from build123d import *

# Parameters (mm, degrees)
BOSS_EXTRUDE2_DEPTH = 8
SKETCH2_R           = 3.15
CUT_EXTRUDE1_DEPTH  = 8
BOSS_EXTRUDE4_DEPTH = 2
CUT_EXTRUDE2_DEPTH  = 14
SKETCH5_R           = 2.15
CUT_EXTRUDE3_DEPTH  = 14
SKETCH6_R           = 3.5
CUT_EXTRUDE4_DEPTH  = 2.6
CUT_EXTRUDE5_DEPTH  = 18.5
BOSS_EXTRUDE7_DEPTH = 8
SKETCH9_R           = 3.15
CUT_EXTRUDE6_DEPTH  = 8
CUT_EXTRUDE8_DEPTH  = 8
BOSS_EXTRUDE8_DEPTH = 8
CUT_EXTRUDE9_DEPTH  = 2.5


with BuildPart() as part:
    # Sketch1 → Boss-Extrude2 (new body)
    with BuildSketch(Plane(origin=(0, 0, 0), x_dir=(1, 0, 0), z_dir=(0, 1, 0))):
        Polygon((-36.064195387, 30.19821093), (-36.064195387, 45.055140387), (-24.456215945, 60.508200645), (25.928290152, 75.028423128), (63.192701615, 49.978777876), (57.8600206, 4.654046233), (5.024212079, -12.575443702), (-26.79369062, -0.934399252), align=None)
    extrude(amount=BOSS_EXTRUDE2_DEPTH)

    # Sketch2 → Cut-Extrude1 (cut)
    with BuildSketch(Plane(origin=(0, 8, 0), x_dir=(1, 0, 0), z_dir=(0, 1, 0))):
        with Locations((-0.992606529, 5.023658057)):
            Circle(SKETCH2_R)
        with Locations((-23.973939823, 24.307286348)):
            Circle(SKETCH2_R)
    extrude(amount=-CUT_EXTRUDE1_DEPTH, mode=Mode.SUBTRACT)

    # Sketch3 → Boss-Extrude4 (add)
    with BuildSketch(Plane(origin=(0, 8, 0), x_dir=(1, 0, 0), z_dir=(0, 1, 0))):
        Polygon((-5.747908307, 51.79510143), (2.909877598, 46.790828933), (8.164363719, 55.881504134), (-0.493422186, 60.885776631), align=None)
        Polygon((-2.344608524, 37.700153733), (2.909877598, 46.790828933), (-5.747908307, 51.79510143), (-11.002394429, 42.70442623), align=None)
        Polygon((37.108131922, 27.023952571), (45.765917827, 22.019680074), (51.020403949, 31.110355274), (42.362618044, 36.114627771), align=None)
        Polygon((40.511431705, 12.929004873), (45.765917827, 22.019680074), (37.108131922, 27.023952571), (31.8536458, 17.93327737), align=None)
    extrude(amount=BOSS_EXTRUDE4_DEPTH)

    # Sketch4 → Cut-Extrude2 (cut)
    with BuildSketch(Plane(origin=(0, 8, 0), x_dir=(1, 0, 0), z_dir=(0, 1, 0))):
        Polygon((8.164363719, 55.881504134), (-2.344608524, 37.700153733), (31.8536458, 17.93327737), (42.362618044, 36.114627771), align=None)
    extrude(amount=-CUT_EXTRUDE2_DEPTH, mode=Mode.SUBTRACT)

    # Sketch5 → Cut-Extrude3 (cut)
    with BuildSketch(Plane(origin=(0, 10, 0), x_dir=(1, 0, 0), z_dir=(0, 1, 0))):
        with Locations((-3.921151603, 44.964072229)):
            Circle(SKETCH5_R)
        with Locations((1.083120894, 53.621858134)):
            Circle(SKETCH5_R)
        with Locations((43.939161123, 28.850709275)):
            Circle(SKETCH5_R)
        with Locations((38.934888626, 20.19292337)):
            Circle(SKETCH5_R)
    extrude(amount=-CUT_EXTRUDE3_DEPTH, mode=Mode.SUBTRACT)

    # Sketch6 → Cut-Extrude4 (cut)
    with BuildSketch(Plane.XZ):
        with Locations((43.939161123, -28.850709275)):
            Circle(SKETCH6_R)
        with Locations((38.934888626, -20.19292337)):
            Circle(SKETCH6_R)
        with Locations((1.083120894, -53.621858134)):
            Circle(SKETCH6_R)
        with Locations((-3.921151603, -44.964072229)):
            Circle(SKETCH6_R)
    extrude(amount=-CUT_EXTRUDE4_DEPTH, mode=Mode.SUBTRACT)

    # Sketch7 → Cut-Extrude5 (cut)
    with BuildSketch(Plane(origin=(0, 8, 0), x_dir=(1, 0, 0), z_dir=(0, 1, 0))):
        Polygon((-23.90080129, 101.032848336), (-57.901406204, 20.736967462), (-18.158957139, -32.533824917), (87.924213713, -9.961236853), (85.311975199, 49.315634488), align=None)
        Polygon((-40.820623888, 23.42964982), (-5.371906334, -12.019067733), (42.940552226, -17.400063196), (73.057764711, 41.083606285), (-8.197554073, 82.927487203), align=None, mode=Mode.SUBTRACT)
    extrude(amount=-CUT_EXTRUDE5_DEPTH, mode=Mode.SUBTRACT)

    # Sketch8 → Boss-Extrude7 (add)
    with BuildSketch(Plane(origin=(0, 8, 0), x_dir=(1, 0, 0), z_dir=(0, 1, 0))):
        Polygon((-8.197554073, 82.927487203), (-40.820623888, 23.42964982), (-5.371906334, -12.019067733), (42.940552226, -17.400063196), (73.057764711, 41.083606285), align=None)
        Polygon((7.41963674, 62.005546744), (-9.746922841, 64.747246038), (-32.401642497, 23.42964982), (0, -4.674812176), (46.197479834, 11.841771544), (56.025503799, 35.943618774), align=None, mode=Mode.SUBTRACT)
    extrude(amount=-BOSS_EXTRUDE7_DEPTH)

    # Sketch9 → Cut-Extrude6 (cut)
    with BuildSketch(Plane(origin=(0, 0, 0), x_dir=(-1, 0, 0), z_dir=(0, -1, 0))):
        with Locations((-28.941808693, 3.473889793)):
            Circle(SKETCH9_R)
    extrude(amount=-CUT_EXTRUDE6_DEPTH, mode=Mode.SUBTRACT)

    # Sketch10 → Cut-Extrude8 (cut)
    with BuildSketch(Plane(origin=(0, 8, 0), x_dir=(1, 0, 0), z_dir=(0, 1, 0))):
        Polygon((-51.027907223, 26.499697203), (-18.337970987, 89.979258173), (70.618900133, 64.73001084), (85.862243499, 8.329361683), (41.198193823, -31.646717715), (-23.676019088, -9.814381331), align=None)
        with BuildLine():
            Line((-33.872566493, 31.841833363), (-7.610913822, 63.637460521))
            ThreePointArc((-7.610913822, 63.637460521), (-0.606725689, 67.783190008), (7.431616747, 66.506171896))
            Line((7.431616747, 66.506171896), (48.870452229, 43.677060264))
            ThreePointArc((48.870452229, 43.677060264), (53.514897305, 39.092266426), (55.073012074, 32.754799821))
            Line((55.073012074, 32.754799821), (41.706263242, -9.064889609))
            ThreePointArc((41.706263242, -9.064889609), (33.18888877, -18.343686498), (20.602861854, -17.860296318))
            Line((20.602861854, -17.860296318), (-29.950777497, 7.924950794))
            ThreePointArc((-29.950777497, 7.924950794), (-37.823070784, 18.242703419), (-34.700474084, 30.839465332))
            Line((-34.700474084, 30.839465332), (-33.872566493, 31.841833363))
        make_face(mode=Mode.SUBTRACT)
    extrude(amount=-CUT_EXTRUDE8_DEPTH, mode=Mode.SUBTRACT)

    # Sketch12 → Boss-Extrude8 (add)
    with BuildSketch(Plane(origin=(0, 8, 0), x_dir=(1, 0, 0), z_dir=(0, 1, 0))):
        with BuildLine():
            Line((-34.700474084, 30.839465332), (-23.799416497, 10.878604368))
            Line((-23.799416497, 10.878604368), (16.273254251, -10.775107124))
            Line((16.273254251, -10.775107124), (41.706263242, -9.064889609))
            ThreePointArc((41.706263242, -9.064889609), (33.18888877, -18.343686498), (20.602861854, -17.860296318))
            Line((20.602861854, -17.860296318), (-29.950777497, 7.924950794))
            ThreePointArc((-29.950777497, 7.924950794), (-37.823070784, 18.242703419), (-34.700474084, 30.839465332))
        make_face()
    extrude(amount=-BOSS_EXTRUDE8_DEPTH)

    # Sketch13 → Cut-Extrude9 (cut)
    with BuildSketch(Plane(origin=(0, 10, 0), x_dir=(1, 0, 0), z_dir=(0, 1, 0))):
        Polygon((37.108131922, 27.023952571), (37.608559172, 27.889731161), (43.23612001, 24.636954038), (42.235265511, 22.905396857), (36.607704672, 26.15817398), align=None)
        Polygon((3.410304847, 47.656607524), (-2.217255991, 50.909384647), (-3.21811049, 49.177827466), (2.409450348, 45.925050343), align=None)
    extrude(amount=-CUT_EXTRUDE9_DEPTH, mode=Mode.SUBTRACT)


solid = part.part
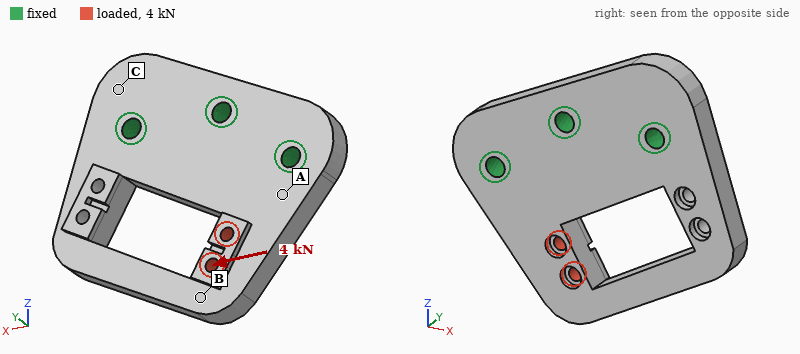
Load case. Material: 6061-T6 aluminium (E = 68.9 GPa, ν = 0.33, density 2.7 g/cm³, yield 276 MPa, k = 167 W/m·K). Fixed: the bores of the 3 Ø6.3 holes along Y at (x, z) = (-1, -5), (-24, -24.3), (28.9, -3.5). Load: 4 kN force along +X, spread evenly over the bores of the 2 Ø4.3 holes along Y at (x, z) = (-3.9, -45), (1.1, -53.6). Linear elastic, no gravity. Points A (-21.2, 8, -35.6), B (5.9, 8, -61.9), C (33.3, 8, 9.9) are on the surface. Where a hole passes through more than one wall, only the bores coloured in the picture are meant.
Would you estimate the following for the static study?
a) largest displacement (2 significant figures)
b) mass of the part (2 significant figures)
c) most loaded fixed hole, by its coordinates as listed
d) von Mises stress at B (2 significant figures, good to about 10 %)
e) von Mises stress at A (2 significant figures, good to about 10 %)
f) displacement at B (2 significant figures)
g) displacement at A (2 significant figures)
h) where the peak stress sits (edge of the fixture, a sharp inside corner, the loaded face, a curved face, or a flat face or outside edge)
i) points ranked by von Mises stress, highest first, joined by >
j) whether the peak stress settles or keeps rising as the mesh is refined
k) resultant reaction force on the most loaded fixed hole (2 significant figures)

55 µm
94 g
(-24, -24.3)
20 MPa
34 MPa
51 µm
9.0 µm
a sharp inside corner
A > B > C
keeps rising
4.0 kN
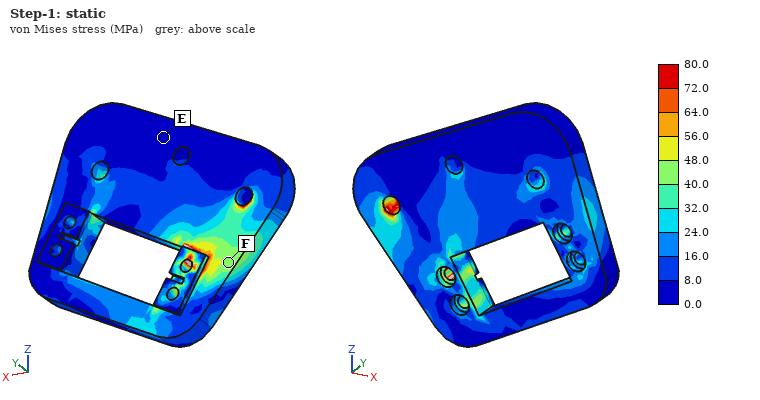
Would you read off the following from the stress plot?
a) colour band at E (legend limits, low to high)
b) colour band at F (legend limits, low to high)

0.0 to 8.0 MPa
40.0 to 48.0 MPa
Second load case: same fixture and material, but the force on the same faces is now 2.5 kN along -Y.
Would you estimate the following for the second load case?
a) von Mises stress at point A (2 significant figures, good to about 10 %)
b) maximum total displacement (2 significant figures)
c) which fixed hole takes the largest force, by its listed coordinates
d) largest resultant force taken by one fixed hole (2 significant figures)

120 MPa
0.45 mm
(-24, -24.3)
2.1 kN
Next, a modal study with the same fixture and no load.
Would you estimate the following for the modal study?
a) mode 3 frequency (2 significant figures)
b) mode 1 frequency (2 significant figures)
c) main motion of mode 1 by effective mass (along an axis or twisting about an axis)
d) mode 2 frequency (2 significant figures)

7700 Hz
2600 Hz
along Y
4700 Hz
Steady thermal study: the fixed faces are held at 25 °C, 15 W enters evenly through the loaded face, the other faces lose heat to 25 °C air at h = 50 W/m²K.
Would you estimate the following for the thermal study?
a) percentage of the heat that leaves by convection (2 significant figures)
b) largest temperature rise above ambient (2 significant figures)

12 %
13 K
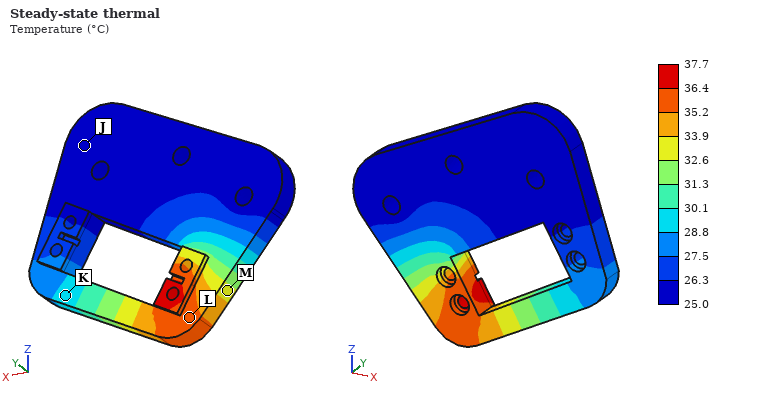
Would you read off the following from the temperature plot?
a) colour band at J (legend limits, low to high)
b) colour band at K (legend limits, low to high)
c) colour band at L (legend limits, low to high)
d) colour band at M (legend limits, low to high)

25.0 to 26.3 °C
28.8 to 30.1 °C
35.2 to 36.4 °C
32.6 to 33.9 °C
